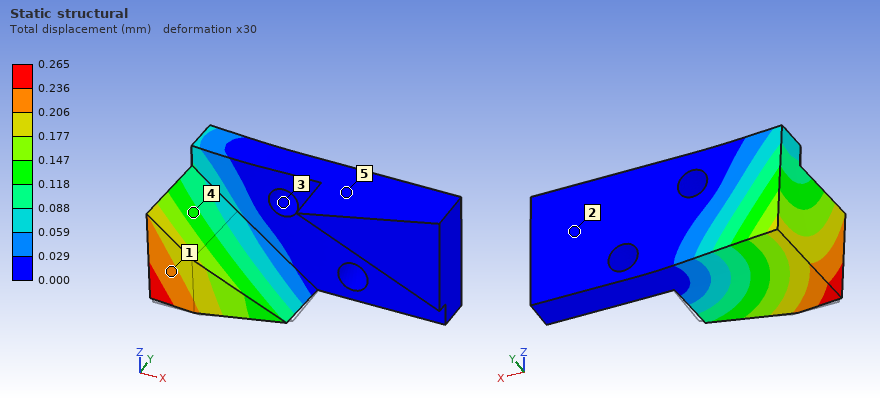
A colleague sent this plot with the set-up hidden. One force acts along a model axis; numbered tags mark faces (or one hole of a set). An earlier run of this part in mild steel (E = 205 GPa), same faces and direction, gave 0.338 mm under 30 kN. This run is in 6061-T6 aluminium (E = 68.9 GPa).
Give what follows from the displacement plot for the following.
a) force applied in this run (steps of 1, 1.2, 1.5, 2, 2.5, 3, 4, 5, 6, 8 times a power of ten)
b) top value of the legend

8 kN
0.265 mm
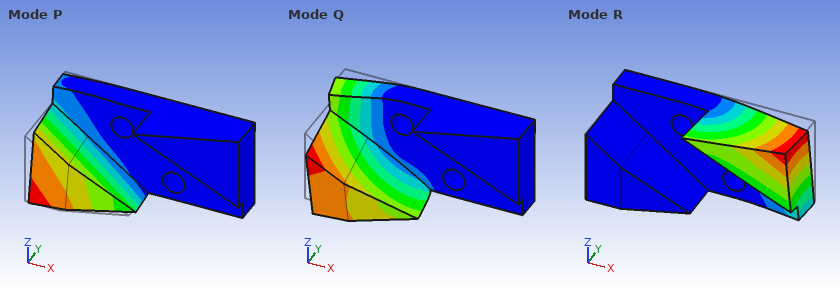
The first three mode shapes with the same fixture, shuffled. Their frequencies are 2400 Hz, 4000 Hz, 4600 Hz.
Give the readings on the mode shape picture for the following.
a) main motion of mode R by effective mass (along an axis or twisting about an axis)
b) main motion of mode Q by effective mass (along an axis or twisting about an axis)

along Y
along Z
